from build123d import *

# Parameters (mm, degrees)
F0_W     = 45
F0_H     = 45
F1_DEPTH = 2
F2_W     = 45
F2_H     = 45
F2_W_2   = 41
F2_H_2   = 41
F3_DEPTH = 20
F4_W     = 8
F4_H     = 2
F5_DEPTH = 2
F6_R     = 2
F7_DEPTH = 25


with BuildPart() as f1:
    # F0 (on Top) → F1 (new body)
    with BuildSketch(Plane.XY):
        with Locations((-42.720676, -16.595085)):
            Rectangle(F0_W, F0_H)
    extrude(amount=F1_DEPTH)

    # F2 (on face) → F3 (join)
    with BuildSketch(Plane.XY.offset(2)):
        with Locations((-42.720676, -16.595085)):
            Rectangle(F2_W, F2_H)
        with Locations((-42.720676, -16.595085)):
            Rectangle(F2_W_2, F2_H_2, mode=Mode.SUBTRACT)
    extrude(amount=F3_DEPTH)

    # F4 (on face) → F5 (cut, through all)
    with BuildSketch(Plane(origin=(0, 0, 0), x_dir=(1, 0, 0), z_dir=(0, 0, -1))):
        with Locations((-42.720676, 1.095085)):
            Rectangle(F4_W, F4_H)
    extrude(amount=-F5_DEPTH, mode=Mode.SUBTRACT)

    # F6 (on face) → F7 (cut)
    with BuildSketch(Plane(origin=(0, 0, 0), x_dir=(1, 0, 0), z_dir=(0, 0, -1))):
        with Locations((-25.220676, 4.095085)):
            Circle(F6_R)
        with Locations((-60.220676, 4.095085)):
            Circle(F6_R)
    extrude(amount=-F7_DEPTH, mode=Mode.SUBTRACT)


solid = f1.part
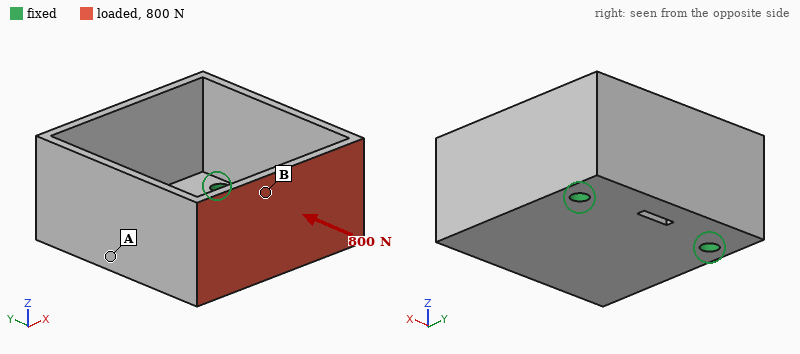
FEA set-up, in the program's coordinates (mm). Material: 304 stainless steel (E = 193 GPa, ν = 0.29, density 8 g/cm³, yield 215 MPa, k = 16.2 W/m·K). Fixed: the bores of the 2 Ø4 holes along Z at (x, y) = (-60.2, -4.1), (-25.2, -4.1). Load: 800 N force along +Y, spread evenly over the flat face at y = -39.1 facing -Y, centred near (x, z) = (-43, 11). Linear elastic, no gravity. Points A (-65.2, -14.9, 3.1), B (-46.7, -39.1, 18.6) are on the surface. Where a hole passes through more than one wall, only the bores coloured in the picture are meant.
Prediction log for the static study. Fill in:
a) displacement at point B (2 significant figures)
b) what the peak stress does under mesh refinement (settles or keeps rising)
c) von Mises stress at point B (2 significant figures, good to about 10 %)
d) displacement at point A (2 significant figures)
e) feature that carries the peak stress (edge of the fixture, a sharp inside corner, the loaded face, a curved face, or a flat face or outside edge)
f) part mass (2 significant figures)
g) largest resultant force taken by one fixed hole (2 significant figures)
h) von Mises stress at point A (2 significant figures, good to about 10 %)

0.12 mm
keeps rising
61 MPa
0.023 mm
edge of the fixture
87 g
400 N
24 MPa
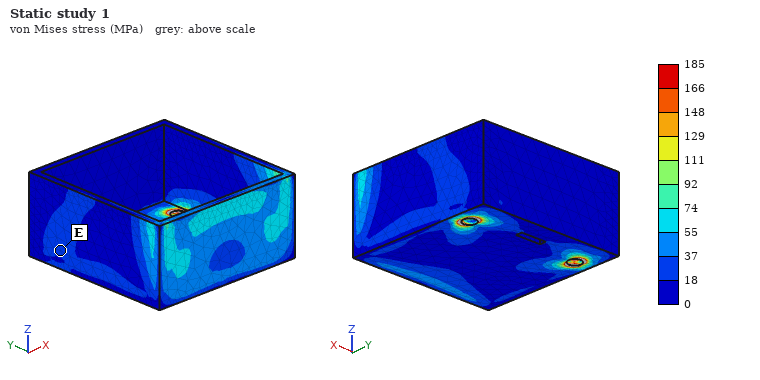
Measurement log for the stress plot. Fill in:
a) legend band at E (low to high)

18 to 37 MPa
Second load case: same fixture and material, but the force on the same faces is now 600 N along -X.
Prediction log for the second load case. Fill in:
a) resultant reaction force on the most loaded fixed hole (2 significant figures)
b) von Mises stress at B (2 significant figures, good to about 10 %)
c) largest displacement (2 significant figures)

670 N
24 MPa
85 µm
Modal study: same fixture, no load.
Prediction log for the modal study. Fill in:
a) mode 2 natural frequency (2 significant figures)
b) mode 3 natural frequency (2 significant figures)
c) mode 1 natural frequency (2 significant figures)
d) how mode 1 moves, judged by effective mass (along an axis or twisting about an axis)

2200 Hz
5200 Hz
1500 Hz
along Z
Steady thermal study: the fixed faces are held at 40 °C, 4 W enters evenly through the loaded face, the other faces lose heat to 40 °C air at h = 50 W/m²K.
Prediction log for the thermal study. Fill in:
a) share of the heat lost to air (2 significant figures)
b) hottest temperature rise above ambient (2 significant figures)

88 %
28 K
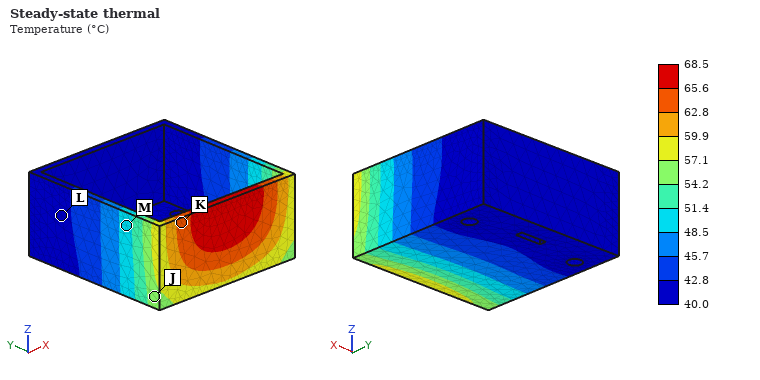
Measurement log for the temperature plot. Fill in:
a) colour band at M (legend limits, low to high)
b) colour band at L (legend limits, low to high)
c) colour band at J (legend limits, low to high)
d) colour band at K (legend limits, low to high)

48.5 to 51.4 °C
40.0 to 42.8 °C
54.2 to 57.1 °C
62.8 to 65.6 °C
